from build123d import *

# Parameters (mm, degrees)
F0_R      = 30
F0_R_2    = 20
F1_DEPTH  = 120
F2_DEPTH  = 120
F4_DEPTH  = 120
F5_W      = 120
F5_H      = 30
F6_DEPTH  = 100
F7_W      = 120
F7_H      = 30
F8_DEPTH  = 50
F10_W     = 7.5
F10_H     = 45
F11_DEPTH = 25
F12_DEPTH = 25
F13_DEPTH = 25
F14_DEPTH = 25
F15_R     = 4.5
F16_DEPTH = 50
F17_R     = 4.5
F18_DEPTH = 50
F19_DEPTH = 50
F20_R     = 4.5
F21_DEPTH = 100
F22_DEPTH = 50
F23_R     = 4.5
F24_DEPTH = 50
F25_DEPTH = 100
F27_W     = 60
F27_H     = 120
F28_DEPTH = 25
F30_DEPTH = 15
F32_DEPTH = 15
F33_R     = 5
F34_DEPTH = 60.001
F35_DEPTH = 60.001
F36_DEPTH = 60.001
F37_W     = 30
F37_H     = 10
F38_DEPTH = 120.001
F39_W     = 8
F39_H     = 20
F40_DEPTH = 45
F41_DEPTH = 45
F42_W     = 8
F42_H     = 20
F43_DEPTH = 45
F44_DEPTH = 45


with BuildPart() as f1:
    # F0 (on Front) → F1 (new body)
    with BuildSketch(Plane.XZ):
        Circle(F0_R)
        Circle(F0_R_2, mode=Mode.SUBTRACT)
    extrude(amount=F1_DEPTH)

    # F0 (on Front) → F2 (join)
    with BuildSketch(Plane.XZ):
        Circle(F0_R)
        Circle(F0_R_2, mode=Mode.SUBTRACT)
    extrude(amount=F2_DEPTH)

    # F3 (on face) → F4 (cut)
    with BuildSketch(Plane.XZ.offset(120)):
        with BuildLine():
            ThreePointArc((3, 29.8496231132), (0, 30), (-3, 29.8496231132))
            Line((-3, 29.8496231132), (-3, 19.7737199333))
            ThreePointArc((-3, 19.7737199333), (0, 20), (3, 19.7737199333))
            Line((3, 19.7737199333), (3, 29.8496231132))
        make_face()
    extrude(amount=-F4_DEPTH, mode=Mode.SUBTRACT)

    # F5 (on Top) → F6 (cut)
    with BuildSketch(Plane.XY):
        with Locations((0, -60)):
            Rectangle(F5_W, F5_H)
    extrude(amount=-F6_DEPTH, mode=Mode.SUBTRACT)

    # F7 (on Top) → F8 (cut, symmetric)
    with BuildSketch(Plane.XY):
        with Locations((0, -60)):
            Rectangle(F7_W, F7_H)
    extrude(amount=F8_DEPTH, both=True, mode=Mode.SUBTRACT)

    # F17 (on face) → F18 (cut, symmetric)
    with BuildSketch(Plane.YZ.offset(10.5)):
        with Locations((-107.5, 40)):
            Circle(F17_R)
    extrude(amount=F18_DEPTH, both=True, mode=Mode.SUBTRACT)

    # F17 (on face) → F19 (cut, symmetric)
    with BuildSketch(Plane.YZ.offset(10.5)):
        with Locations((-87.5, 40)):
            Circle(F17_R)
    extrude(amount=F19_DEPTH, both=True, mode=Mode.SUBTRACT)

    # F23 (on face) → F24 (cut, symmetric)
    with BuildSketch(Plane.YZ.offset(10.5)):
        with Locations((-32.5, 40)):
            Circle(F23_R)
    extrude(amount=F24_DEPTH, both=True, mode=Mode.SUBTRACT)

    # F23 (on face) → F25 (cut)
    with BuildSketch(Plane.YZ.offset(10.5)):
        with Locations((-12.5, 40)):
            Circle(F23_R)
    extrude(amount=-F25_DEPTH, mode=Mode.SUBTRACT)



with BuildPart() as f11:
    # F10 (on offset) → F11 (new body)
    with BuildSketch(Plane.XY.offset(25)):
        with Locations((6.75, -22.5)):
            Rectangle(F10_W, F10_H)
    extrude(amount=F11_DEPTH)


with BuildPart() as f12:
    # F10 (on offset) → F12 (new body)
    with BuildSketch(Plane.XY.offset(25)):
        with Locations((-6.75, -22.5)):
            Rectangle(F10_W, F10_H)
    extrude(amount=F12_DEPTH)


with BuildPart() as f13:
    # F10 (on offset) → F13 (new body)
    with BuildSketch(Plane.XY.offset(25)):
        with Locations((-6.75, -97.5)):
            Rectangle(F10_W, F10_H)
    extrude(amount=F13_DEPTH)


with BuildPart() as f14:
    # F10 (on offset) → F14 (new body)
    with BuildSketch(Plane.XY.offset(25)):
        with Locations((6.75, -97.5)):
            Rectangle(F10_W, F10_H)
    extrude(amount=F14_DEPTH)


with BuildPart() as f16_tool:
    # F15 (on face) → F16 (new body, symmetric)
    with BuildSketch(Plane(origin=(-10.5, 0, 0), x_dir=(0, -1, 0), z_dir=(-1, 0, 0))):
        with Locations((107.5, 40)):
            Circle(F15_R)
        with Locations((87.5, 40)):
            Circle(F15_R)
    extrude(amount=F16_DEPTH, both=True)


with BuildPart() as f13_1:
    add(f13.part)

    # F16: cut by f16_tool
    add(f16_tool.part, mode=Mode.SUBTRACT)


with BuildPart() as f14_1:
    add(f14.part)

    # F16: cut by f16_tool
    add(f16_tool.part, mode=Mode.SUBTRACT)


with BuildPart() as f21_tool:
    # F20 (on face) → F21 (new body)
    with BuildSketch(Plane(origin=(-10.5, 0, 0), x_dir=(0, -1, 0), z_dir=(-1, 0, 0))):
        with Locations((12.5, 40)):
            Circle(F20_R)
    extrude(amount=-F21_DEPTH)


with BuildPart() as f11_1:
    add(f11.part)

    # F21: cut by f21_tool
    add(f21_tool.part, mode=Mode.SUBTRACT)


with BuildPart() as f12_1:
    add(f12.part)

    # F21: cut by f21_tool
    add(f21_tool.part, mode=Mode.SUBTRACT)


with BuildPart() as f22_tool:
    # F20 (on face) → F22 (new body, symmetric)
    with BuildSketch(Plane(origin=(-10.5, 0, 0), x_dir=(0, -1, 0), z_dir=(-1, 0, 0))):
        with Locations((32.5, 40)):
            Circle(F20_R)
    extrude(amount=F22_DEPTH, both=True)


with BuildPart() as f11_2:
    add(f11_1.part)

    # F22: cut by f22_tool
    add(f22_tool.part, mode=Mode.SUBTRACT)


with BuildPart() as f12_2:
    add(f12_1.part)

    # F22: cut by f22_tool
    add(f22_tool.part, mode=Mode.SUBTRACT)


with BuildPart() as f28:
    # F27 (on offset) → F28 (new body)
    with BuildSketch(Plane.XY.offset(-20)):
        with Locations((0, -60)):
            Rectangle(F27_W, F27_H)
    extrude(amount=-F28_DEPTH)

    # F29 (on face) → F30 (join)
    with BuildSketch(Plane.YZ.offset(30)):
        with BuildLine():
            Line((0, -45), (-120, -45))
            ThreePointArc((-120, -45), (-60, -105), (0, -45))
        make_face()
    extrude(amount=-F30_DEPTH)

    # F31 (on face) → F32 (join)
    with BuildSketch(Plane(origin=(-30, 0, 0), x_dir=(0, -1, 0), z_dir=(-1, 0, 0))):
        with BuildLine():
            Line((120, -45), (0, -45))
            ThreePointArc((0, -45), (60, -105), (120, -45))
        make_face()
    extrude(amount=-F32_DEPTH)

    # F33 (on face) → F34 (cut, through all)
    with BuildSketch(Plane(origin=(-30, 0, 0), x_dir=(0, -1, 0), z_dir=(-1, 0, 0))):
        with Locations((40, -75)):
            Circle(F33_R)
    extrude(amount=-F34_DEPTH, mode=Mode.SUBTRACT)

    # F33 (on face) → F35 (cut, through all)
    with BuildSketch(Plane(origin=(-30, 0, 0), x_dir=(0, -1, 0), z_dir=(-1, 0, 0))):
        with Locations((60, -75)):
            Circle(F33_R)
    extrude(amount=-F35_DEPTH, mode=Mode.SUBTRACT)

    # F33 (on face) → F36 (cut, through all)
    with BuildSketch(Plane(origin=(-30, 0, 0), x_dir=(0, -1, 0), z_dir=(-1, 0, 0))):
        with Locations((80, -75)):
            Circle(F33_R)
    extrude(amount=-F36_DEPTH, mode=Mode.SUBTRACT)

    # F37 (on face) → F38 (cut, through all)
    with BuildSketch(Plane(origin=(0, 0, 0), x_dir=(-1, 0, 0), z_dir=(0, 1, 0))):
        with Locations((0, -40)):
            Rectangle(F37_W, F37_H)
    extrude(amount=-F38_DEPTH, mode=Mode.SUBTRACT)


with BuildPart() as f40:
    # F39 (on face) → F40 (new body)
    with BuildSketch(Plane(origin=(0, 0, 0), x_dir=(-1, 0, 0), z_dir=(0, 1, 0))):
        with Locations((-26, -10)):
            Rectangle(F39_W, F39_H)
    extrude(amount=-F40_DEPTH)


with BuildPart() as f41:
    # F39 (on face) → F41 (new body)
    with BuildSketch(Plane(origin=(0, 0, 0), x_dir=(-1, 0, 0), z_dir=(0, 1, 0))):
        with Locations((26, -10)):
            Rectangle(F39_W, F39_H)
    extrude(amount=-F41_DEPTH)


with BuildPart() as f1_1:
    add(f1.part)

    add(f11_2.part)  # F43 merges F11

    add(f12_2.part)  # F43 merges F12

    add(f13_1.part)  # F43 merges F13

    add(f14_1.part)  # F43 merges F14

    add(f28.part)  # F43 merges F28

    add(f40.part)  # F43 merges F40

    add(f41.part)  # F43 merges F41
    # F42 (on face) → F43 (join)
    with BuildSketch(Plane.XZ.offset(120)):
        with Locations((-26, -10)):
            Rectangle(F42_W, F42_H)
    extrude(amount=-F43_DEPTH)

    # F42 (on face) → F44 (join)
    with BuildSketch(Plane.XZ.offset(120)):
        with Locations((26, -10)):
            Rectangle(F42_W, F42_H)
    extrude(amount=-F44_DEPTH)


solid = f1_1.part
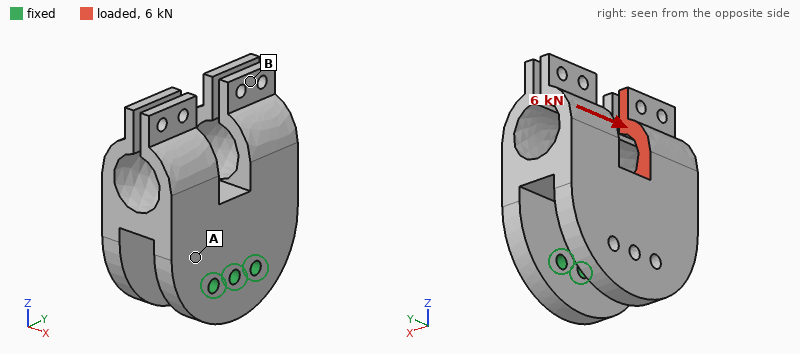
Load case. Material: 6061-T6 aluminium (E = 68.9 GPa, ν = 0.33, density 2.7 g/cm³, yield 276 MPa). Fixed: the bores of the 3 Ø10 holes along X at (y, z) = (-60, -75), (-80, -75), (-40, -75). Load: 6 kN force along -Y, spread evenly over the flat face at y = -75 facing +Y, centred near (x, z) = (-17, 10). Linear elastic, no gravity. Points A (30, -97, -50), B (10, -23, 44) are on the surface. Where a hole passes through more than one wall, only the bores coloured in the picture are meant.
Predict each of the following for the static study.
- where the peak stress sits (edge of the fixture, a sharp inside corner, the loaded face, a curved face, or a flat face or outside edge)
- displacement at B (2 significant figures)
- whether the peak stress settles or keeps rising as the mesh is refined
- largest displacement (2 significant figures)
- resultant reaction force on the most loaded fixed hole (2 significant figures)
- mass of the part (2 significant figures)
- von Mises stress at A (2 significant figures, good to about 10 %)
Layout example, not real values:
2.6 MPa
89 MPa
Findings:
edge of the fixture
0.082 mm
keeps rising
0.29 mm
11 kN
1.2 kg
9.9 MPa
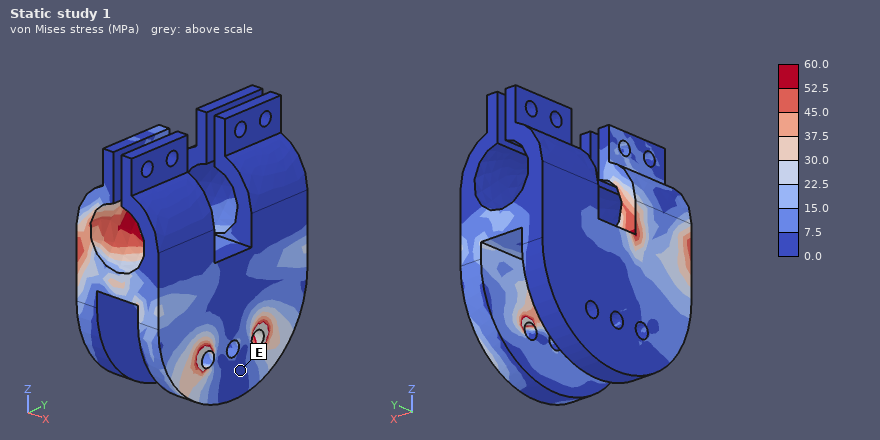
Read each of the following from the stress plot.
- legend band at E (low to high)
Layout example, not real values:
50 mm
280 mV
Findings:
0.0 to 7.5 MPa
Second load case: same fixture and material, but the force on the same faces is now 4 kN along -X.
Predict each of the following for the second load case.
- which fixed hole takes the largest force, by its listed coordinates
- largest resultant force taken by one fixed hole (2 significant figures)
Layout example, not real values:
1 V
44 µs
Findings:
(-80, -75)
2.0 kN
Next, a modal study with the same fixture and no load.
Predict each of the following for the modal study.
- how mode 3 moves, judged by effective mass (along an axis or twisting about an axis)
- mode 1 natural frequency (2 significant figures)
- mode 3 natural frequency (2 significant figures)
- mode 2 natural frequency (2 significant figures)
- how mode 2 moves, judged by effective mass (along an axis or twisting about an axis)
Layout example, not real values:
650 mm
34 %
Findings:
along X
590 Hz
1500 Hz
1000 Hz
along Y
